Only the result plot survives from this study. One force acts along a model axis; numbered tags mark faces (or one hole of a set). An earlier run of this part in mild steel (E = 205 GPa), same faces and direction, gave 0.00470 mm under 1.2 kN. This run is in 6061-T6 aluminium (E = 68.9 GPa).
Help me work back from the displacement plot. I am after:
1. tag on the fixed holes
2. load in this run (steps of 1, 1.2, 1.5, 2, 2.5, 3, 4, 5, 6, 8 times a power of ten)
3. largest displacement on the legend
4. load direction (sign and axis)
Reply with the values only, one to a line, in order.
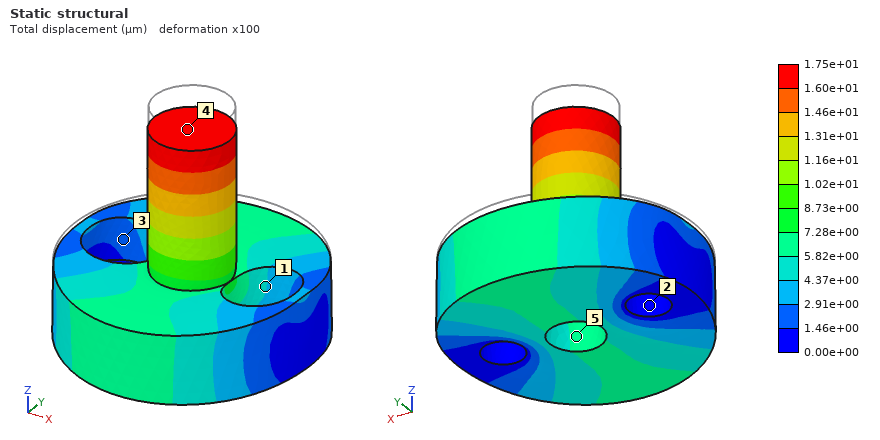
2
1.5 kN
1.75e+01 µm
-Z
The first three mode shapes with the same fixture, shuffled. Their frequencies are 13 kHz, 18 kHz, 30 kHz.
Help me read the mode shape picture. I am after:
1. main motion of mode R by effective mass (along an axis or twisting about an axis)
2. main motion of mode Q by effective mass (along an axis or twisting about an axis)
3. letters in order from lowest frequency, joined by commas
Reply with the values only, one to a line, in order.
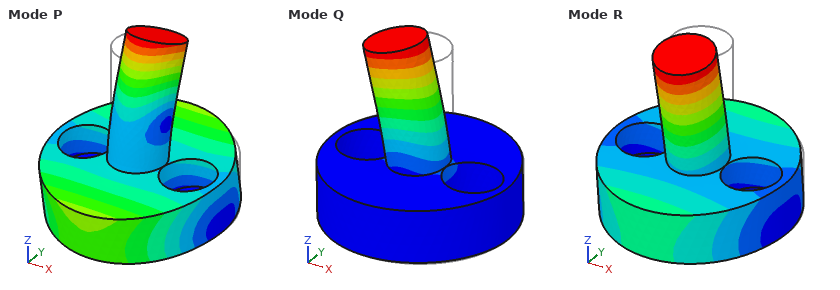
along Y
along X
R, Q, P
